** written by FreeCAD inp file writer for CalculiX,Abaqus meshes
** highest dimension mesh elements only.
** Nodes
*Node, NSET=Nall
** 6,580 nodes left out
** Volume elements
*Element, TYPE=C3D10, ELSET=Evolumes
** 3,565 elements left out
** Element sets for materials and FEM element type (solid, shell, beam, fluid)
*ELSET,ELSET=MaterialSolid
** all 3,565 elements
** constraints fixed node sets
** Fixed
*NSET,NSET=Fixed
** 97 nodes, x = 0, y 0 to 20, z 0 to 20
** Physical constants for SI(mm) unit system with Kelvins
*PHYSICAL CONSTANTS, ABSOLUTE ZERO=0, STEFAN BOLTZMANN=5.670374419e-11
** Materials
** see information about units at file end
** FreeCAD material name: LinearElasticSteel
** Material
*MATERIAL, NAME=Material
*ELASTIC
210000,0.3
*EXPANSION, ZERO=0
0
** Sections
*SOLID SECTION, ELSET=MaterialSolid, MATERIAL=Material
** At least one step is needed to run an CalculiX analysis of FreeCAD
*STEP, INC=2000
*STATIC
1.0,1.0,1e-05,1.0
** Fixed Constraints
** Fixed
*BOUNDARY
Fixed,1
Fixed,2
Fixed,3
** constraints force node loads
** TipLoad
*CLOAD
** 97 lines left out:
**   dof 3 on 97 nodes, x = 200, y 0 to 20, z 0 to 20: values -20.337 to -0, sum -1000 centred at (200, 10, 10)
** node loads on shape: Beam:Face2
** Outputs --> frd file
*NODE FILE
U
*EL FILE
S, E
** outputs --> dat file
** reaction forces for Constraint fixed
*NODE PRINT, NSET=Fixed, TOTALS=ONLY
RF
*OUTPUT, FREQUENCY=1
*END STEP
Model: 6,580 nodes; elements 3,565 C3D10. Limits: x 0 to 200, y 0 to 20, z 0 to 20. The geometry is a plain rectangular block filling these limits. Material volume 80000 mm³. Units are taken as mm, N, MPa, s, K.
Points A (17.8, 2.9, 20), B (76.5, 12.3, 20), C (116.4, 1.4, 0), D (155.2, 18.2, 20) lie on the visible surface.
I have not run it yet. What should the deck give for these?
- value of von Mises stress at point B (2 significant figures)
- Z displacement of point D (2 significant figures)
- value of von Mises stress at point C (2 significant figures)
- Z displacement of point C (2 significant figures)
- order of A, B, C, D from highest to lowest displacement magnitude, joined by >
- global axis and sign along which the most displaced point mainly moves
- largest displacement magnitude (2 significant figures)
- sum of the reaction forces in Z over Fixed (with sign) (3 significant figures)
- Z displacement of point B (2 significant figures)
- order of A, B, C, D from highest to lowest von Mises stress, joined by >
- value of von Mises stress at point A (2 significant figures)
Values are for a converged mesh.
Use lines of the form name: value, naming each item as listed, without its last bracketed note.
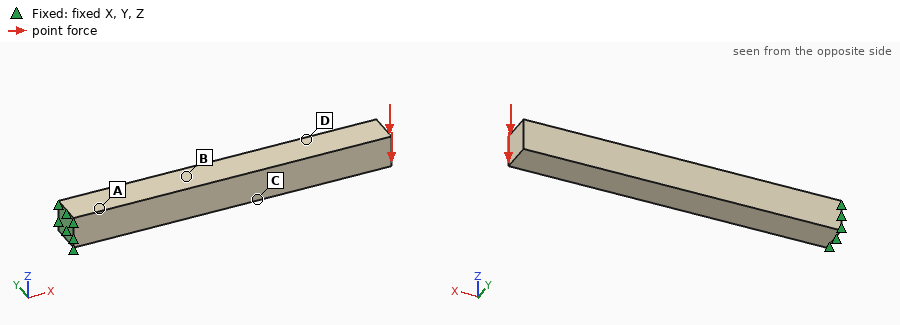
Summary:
value of von Mises stress at point B: 92 MPa
Z displacement of point D: -0.64 mm
value of von Mises stress at point C: 63 MPa
Z displacement of point C: -0.39 mm
order of A, B, C, D from highest to lowest displacement magnitude, joined by >: D > C > B > A
global axis and sign along which the most displaced point mainly moves: -Z
largest displacement magnitude: 0.96 mm
sum of the reaction forces in Z over Fixed (with sign): 1000 N
Z displacement of point B: -0.18 mm
order of A, B, C, D from highest to lowest von Mises stress, joined by >: A > B > C > D
value of von Mises stress at point A: 140 MPa
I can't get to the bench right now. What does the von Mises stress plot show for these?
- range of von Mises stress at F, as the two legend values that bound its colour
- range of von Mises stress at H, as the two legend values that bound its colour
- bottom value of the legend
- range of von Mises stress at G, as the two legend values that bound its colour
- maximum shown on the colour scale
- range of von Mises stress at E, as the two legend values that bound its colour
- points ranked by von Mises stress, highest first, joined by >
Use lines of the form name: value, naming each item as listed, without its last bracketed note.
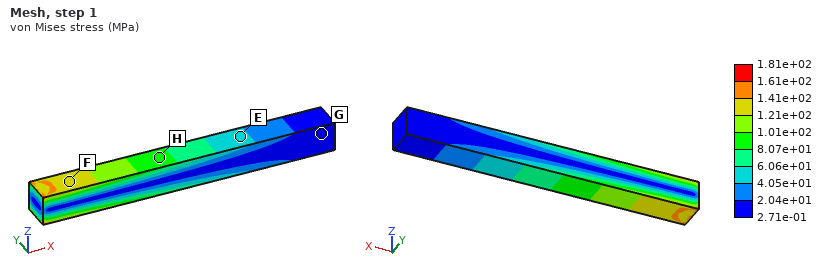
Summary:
range of von Mises stress at F, as the two legend values that bound its colour: 1.21e+02 to 1.41e+02 MPa
range of von Mises stress at H, as the two legend values that bound its colour: 8.07e+01 to 1.01e+02 MPa
bottom value of the legend: 2.71e-01 MPa
range of von Mises stress at G, as the two legend values that bound its colour: 2.71e-01 to 2.04e+01 MPa
maximum shown on the colour scale: 1.81e+02 MPa
range of von Mises stress at E, as the two legend values that bound its colour: 4.05e+01 to 6.06e+01 MPa
points ranked by von Mises stress, highest first, joined by >: F > H > E > G
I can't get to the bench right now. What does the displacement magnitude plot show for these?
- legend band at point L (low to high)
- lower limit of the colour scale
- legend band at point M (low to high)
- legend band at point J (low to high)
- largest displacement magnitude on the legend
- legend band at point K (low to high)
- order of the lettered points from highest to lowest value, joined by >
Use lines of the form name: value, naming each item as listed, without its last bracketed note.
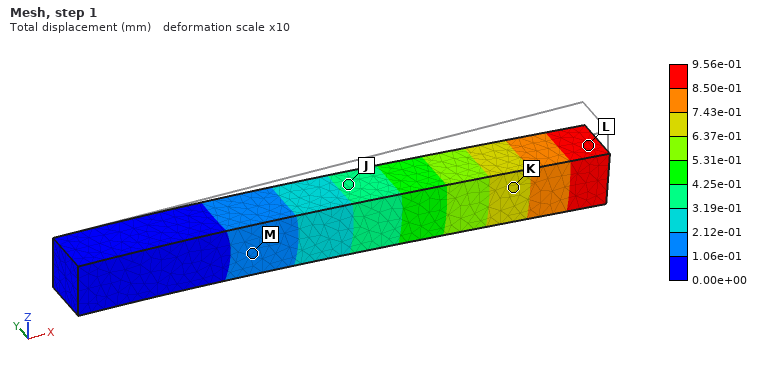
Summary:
legend band at point L: 8.50e-01 to 9.56e-01 mm
lower limit of the colour scale: 0.00e+00 mm
legend band at point M: 1.06e-01 to 2.12e-01 mm
legend band at point J: 3.19e-01 to 4.25e-01 mm
largest displacement magnitude on the legend: 9.56e-01 mm
legend band at point K: 6.37e-01 to 7.43e-01 mm
order of the lettered points from highest to lowest value, joined by >: L > K > J > M
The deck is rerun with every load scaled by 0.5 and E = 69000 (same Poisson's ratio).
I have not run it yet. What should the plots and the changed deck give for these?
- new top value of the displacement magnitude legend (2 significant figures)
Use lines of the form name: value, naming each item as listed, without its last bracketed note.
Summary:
new top value of the displacement magnitude legend: 1.5 mm
